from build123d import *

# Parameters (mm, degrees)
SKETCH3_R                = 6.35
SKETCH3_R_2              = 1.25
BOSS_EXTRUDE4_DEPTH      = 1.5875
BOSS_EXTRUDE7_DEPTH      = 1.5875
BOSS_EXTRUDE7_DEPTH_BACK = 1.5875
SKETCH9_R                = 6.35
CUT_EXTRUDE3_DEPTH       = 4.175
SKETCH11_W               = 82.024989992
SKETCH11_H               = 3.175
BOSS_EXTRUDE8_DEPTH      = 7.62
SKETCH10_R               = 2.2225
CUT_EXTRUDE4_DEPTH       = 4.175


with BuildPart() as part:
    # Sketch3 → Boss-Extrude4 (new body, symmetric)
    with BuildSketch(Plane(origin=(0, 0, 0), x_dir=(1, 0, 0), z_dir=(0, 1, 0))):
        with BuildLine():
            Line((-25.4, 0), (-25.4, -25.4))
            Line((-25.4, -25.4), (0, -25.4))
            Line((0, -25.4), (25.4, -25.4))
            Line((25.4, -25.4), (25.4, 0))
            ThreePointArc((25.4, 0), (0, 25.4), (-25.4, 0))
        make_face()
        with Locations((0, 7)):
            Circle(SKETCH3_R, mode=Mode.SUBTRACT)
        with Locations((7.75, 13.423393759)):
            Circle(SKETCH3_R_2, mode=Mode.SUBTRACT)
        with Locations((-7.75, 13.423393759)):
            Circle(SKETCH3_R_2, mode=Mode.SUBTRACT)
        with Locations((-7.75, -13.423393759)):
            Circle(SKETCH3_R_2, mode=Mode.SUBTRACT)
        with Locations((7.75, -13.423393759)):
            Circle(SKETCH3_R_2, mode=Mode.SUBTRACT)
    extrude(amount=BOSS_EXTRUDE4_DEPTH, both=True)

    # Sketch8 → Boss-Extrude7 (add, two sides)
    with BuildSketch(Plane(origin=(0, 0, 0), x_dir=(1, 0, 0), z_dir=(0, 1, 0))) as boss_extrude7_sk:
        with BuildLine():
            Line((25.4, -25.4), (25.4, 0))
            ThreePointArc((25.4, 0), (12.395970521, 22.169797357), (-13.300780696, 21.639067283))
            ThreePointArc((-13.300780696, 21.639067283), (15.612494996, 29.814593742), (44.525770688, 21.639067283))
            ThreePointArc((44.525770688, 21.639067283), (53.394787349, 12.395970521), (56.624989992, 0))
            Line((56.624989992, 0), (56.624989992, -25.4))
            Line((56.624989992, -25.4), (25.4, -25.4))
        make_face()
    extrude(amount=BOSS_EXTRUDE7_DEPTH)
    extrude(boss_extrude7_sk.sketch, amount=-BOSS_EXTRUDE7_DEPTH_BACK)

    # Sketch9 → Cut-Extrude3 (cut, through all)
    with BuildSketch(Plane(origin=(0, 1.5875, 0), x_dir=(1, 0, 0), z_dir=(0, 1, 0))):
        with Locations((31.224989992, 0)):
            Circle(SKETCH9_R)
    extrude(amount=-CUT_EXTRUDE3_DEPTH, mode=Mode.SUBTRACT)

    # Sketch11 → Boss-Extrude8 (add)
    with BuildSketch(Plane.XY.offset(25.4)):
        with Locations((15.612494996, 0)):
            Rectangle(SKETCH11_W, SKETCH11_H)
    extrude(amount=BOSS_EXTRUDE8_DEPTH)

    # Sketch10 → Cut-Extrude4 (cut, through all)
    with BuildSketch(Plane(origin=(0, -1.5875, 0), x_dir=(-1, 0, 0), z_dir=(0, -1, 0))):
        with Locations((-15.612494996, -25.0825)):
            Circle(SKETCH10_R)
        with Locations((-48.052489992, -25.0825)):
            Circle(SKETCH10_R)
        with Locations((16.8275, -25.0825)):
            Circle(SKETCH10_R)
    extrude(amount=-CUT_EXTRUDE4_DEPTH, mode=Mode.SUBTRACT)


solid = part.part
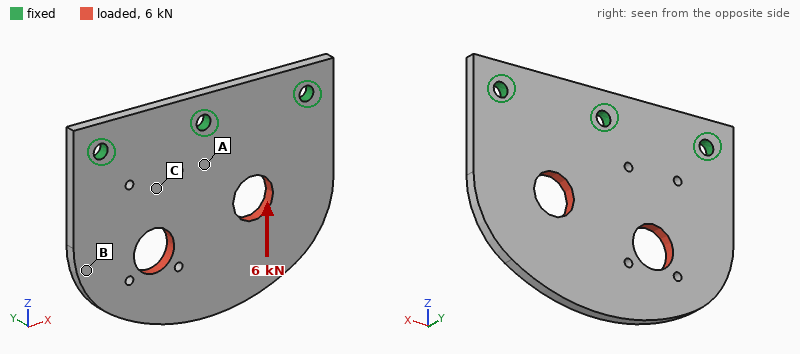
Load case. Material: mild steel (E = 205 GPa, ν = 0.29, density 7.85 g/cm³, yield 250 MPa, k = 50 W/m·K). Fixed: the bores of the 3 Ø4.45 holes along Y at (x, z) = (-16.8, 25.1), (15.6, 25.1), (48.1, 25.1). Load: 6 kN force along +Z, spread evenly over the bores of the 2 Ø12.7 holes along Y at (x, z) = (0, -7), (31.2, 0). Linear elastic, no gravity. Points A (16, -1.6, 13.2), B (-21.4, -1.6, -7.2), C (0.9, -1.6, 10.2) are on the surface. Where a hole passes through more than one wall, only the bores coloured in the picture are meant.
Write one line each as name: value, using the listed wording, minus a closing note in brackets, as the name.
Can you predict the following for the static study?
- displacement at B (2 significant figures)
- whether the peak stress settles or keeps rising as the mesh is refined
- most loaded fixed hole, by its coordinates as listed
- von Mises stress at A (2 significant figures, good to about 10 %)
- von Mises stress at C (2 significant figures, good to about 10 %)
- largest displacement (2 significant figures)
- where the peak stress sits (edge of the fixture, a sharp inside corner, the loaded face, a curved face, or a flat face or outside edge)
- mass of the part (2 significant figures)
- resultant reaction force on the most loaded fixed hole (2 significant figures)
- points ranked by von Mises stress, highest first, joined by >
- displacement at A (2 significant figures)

displacement at B: 3.0 µm
whether the peak stress settles or keeps rising as the mesh is refined: keeps rising
most loaded fixed hole, by its coordinates as listed: (15.6, 25.1)
von Mises stress at A: 37 MPa
von Mises stress at C: 21 MPa
largest displacement: 7.4 µm
where the peak stress sits: edge of the fixture
mass of the part: 110 g
resultant reaction force on the most loaded fixed hole: 2.5 kN
points ranked by von Mises stress, highest first, joined by >: A > C > B
displacement at A: 2.6 µm
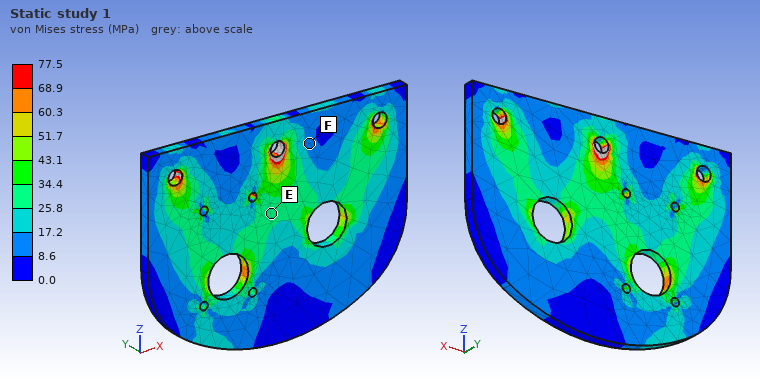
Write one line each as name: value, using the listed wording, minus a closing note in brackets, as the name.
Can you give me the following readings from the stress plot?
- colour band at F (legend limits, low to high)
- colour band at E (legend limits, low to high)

colour band at F: 8.6 to 17.2 MPa
colour band at E: 25.8 to 34.4 MPa
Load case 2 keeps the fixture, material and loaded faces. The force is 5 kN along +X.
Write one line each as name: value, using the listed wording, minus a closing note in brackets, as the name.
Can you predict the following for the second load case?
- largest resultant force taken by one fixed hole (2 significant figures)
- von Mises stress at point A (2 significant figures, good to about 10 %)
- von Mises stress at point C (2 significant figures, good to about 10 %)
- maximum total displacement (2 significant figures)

largest resultant force taken by one fixed hole: 2.5 kN
von Mises stress at point A: 35 MPa
von Mises stress at point C: 48 MPa
maximum total displacement: 15 µm
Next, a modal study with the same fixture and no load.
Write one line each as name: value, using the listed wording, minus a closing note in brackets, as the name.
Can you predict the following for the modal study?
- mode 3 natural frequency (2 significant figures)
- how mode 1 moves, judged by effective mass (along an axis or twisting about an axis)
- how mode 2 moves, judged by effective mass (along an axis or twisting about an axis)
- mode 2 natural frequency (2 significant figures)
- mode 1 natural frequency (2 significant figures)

mode 3 natural frequency: 4400 Hz
how mode 1 moves, judged by effective mass: along Y
how mode 2 moves, judged by effective mass: twisting about Z
mode 2 natural frequency: 2200 Hz
mode 1 natural frequency: 1000 Hz
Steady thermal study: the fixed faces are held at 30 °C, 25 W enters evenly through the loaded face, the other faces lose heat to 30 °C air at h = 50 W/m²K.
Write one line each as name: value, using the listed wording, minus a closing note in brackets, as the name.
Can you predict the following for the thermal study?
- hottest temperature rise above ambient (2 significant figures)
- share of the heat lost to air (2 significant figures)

hottest temperature rise above ambient: 51 K
share of the heat lost to air: 44 %
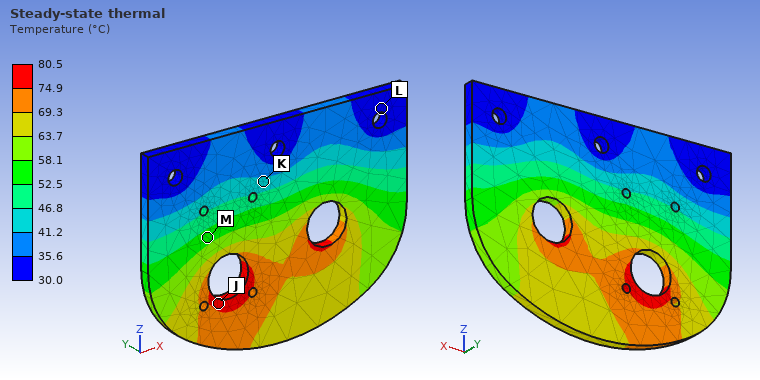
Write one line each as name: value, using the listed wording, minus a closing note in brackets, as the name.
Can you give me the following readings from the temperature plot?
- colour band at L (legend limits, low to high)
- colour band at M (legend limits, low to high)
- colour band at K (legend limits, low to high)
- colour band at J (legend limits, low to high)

colour band at L: 30.0 to 35.6 °C
colour band at M: 52.5 to 58.1 °C
colour band at K: 41.2 to 46.8 °C
colour band at J: 74.9 to 80.5 °C
